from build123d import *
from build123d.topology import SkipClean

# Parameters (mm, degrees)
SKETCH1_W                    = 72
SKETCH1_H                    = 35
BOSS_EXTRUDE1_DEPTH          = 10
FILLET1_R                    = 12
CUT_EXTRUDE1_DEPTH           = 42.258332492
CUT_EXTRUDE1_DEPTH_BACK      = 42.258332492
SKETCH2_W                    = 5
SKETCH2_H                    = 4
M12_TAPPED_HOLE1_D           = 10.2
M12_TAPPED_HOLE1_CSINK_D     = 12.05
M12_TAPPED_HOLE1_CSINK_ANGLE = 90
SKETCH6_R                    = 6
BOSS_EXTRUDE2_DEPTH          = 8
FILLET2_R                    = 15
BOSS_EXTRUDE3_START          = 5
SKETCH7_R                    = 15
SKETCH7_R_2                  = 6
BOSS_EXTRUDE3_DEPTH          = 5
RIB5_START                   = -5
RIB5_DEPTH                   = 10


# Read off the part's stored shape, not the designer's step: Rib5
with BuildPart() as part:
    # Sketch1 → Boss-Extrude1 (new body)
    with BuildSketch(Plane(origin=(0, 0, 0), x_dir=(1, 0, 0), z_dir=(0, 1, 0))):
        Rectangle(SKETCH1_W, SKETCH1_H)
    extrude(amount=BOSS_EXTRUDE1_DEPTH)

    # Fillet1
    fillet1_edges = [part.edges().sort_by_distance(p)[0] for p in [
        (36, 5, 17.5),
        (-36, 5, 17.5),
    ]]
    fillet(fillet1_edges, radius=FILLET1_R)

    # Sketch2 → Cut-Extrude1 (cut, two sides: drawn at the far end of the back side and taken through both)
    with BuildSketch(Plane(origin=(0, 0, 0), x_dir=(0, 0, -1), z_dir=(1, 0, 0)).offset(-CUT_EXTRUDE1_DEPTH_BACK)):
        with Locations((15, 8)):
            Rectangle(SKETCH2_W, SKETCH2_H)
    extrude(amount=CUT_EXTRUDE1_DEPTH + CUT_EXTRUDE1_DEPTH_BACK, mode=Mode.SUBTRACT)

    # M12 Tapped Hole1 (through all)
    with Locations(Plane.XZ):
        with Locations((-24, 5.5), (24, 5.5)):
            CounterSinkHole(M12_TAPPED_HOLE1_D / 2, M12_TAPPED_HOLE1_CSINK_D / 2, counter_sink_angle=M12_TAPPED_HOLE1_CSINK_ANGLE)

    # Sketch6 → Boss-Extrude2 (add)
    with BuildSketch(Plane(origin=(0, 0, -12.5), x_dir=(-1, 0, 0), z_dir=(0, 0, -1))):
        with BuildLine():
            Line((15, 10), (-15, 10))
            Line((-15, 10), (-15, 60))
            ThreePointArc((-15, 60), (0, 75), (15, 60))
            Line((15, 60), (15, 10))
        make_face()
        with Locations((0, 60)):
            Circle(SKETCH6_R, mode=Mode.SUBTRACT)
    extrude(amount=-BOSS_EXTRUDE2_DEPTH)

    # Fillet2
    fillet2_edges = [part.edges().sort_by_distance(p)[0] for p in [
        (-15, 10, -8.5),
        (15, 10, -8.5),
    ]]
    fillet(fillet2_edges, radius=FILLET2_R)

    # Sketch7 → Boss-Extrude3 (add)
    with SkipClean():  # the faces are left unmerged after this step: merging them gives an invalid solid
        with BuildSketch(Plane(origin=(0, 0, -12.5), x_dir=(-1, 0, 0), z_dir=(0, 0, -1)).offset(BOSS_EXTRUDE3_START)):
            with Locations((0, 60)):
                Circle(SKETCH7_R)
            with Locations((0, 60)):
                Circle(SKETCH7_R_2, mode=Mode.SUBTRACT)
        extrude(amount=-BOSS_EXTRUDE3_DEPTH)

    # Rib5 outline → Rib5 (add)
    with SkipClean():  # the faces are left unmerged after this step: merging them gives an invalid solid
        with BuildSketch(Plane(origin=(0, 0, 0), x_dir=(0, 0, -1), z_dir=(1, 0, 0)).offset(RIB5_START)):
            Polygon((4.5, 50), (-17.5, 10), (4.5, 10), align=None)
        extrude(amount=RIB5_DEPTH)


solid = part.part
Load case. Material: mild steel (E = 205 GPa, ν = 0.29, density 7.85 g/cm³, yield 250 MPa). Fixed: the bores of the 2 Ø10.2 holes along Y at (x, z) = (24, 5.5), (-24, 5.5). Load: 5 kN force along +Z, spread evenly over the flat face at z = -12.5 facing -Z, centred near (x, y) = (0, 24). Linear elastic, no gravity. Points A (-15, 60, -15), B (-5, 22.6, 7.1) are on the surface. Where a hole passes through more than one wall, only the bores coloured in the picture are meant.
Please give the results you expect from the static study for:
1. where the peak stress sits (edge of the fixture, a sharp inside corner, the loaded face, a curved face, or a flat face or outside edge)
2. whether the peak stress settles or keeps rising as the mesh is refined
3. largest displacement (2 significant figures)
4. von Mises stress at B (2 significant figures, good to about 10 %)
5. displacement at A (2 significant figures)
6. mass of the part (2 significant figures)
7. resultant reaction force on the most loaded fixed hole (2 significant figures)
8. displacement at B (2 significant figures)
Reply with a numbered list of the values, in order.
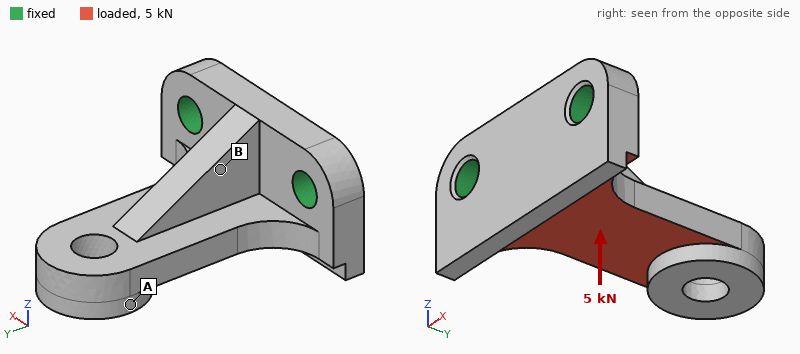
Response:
1. edge of the fixture
2. keeps rising
3. 79 µm
4. 31 MPa
5. 62 µm
6. 340 g
7. 2.5 kN
8. 19 µm
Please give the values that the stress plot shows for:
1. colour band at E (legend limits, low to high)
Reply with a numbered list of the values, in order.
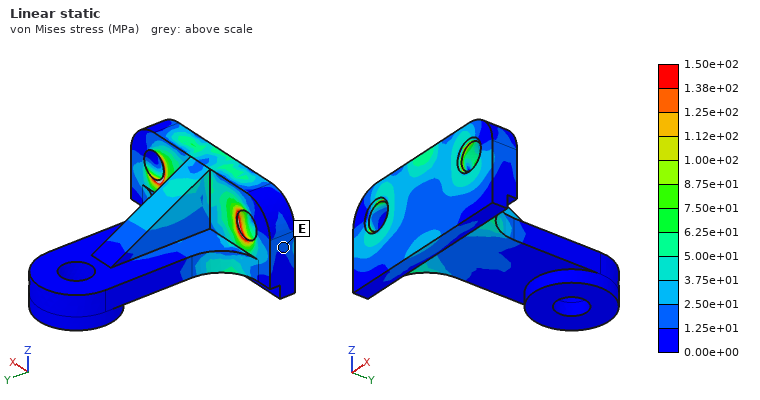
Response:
1. 1.25e+01 to 2.50e+01 MPa
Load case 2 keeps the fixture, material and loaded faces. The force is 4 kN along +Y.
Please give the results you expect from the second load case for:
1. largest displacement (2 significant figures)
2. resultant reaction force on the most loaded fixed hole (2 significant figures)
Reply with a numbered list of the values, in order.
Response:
1. 41 µm
2. 2.0 kN
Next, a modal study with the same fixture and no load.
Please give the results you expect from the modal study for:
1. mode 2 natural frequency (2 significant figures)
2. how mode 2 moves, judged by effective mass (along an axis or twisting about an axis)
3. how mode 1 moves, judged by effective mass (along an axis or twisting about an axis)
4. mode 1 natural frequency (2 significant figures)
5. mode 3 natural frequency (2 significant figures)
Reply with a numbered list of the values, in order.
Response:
1. 4300 Hz
2. along X
3. along Z
4. 2500 Hz
5. 7800 Hz
